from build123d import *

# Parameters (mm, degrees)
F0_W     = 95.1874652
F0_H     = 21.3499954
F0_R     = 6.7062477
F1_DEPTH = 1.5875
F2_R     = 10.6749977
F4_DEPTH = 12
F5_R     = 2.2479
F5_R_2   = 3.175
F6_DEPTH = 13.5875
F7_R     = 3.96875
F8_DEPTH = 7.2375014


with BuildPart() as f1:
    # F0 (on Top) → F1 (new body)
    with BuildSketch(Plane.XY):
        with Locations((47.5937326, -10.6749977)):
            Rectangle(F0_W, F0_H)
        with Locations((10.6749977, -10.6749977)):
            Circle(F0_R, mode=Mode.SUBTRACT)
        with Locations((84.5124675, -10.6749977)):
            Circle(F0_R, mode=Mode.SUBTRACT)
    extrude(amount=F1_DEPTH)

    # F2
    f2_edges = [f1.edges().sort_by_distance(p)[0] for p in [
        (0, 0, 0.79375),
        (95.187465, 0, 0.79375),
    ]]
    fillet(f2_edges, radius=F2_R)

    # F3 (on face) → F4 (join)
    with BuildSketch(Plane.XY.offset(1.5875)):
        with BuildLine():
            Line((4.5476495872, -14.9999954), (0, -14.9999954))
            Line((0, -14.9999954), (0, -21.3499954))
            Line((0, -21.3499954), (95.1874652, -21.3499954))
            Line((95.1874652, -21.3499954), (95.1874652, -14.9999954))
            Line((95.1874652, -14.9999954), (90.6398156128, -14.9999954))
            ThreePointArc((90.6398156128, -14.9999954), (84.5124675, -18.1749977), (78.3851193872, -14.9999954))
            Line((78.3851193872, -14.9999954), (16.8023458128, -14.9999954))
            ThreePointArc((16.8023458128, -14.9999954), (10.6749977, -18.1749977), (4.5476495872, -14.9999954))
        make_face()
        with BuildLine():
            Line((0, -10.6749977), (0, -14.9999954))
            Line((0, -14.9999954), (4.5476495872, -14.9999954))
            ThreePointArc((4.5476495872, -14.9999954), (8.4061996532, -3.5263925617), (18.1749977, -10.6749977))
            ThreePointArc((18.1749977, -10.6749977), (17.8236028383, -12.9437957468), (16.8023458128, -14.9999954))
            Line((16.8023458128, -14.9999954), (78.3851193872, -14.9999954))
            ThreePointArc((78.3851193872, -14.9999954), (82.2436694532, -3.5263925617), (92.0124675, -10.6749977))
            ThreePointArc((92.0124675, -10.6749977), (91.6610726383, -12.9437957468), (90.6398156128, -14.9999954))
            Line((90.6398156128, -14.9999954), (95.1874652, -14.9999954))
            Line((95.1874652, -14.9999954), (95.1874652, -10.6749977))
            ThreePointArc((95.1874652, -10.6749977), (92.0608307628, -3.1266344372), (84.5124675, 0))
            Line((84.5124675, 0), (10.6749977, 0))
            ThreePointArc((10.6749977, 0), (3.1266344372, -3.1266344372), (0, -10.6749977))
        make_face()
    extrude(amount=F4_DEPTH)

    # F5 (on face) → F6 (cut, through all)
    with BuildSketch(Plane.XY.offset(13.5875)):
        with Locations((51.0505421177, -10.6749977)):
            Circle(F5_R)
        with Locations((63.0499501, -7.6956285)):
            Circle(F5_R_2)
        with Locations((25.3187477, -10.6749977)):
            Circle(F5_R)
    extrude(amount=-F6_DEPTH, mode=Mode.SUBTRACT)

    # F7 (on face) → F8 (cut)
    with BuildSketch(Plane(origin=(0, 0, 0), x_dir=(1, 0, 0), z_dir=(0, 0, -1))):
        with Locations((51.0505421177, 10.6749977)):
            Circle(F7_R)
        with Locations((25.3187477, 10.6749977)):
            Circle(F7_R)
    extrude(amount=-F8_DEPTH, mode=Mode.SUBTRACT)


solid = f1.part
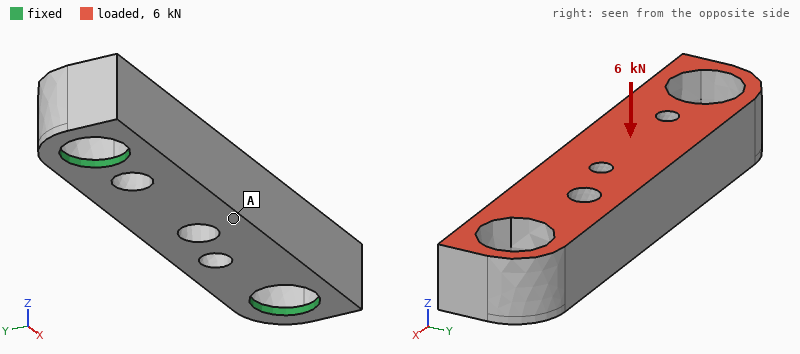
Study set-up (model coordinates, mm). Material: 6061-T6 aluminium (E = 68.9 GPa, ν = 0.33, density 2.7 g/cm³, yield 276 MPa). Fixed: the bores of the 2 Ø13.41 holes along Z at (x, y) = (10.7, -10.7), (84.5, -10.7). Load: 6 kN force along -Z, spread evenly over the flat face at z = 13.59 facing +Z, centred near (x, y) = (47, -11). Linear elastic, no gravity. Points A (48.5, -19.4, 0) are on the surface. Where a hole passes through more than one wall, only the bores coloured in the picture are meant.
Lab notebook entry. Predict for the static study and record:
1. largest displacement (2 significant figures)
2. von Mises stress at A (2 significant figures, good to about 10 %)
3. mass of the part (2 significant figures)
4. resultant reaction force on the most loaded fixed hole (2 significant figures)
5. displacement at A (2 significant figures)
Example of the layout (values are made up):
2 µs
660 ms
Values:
40 µm
29 MPa
56 g
3.8 kN
39 µm
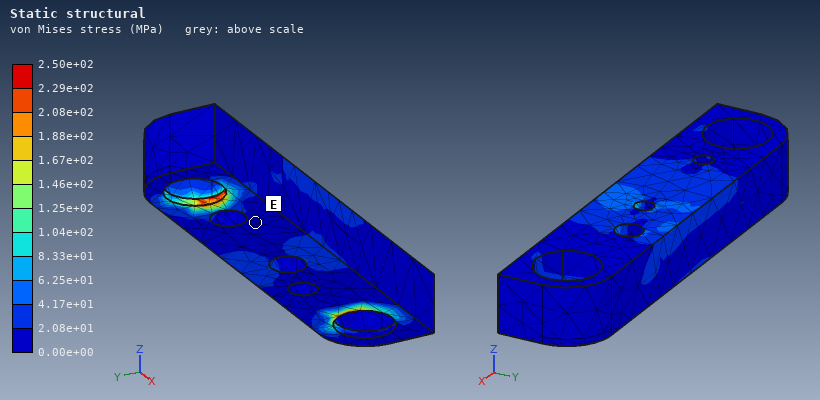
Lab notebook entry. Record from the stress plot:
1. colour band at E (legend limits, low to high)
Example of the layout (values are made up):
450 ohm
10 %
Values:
0.00e+00 to 2.08e+01 MPa
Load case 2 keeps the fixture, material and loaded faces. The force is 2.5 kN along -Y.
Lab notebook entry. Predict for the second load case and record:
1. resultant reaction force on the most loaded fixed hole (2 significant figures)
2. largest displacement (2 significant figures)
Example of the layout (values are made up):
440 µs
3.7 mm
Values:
1.3 kN
40 µm
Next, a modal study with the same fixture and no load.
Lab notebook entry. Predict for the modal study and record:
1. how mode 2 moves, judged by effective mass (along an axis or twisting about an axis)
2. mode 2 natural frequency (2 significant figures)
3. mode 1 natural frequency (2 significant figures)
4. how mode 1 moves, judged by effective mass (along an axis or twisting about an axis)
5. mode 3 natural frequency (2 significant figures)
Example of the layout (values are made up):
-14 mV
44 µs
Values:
along Z
9200 Hz
8400 Hz
along Y
14 kHz
